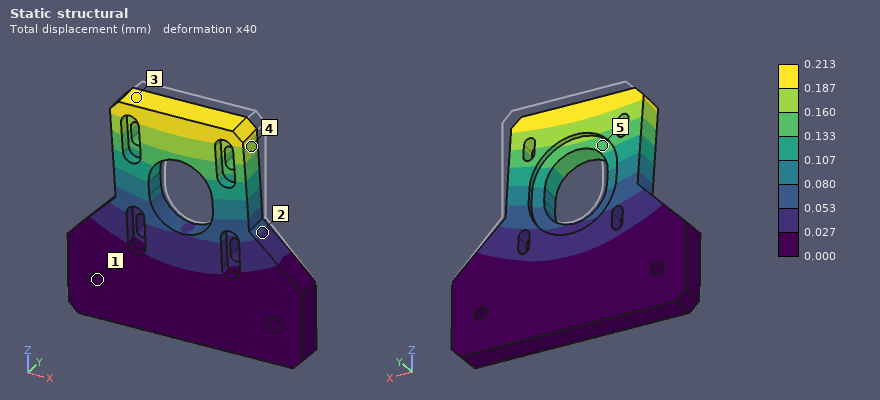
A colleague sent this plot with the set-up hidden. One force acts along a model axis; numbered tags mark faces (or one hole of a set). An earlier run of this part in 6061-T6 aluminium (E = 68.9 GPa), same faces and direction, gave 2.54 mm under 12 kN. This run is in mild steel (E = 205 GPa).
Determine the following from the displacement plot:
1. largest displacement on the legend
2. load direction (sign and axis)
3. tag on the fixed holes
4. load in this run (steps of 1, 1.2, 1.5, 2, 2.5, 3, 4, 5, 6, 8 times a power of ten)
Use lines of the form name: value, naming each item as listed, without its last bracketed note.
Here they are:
largest displacement on the legend: 0.213 mm
load direction: -Y
tag on the fixed holes: 1
load in this run: 3 kN
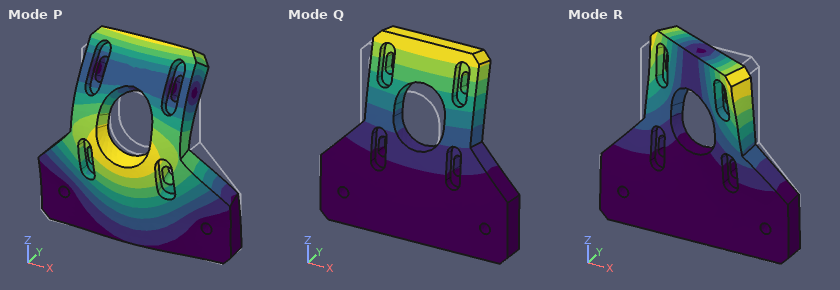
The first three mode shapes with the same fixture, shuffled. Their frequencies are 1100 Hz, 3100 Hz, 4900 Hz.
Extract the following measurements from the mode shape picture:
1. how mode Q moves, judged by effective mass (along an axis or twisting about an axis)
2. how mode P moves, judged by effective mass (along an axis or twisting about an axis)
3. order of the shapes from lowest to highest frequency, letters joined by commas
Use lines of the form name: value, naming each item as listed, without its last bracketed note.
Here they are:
how mode Q moves, judged by effective mass: along Y
how mode P moves, judged by effective mass: along Y
order of the shapes from lowest to highest frequency, letters joined by commas: Q, R, P
